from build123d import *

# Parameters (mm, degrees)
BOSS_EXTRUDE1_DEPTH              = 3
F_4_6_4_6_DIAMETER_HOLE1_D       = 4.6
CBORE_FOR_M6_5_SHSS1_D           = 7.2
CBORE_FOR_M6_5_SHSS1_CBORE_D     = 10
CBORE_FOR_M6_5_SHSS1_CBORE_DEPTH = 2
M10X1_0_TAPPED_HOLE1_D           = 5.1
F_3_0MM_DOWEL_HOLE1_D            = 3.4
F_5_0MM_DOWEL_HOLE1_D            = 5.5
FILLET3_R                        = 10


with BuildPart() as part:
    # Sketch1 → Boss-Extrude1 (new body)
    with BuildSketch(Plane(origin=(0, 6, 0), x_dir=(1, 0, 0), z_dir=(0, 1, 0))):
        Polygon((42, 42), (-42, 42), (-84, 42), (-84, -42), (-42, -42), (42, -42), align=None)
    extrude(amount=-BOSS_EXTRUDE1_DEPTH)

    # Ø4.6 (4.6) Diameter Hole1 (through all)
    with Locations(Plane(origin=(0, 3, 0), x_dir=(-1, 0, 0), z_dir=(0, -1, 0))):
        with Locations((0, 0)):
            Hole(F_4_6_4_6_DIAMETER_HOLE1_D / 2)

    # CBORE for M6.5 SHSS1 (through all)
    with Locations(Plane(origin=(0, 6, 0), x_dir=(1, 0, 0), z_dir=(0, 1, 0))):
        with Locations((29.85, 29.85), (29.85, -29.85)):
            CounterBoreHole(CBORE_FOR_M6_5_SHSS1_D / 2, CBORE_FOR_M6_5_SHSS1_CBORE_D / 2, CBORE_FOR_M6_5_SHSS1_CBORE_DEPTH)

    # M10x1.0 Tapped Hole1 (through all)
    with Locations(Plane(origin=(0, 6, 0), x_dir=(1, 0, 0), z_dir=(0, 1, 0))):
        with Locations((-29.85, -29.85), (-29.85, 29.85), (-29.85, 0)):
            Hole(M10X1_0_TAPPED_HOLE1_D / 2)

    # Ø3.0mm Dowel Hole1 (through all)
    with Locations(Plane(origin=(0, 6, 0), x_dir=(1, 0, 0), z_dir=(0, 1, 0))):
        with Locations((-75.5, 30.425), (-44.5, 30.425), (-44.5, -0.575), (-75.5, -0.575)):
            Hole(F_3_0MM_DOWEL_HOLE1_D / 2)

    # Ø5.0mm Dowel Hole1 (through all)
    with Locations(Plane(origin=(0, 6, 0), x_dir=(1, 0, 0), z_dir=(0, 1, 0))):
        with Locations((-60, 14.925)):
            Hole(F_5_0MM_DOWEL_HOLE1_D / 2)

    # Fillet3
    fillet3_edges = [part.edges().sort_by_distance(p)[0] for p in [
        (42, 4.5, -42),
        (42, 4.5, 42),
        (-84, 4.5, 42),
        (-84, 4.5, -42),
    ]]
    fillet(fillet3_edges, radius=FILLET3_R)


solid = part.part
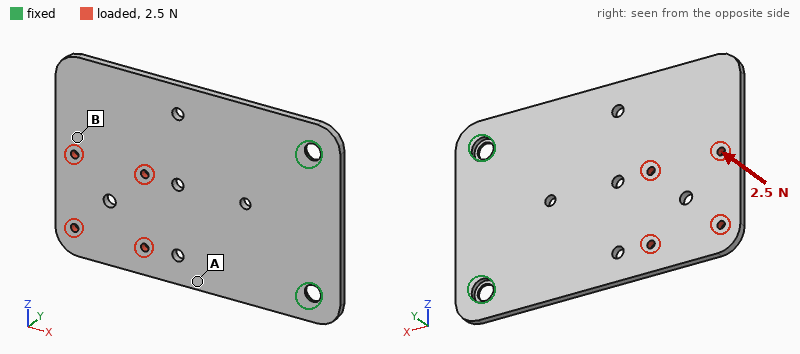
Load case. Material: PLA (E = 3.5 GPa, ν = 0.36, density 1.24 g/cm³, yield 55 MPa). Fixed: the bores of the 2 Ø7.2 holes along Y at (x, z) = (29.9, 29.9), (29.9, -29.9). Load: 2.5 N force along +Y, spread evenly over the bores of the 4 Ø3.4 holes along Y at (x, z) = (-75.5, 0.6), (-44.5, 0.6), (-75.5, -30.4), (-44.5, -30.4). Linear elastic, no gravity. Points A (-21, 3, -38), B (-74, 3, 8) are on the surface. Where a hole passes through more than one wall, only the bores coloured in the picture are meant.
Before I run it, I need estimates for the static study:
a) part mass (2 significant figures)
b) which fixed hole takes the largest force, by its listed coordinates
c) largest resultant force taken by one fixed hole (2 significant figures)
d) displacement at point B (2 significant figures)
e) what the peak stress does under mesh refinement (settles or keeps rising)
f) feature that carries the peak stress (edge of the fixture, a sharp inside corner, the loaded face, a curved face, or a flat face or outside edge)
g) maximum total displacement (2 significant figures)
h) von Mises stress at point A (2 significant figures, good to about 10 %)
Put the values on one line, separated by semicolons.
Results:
38 g; (29.9, -29.9); 3.7 N; 1.5 mm; keeps rising; edge of the fixture; 1.8 mm; 0.84 MPa
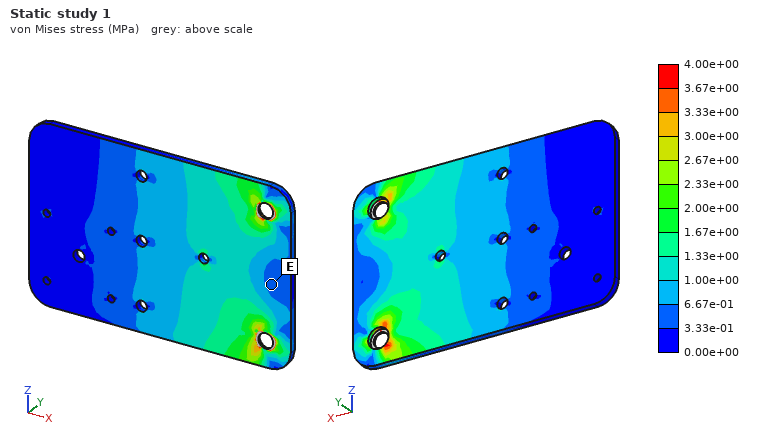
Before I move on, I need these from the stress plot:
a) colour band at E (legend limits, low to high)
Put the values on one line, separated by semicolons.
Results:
3.33e-01 to 6.67e-01 MPa
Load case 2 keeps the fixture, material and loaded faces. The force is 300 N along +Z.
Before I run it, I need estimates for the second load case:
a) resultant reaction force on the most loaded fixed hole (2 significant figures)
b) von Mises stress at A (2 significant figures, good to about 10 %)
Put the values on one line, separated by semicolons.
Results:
460 N; 3.7 MPa
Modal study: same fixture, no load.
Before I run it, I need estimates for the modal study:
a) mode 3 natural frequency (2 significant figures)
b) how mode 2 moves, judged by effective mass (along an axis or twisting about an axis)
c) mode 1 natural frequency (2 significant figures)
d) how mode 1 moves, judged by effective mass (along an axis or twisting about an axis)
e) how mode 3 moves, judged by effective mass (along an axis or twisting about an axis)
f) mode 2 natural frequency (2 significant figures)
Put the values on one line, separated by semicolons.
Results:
350 Hz; twisting about X; 55 Hz; along Y; along Y; 190 Hz
